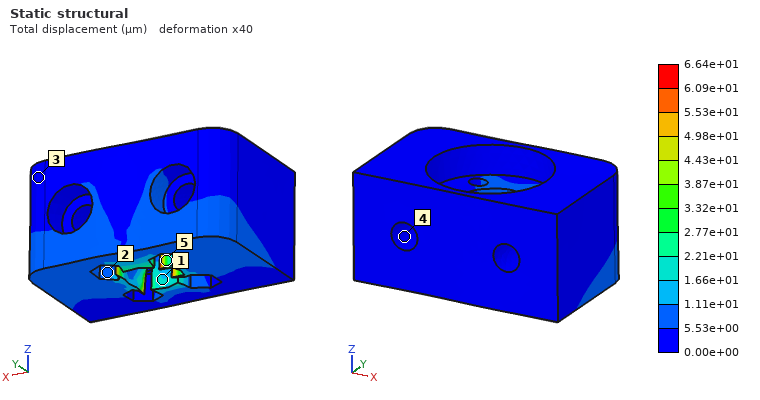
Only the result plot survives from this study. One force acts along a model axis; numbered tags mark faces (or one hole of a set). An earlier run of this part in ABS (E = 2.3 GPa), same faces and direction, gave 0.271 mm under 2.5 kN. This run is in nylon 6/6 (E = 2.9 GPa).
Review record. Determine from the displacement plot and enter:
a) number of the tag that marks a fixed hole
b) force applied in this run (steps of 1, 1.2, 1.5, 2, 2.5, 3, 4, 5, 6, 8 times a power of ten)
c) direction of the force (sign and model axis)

4
800 N
+X
